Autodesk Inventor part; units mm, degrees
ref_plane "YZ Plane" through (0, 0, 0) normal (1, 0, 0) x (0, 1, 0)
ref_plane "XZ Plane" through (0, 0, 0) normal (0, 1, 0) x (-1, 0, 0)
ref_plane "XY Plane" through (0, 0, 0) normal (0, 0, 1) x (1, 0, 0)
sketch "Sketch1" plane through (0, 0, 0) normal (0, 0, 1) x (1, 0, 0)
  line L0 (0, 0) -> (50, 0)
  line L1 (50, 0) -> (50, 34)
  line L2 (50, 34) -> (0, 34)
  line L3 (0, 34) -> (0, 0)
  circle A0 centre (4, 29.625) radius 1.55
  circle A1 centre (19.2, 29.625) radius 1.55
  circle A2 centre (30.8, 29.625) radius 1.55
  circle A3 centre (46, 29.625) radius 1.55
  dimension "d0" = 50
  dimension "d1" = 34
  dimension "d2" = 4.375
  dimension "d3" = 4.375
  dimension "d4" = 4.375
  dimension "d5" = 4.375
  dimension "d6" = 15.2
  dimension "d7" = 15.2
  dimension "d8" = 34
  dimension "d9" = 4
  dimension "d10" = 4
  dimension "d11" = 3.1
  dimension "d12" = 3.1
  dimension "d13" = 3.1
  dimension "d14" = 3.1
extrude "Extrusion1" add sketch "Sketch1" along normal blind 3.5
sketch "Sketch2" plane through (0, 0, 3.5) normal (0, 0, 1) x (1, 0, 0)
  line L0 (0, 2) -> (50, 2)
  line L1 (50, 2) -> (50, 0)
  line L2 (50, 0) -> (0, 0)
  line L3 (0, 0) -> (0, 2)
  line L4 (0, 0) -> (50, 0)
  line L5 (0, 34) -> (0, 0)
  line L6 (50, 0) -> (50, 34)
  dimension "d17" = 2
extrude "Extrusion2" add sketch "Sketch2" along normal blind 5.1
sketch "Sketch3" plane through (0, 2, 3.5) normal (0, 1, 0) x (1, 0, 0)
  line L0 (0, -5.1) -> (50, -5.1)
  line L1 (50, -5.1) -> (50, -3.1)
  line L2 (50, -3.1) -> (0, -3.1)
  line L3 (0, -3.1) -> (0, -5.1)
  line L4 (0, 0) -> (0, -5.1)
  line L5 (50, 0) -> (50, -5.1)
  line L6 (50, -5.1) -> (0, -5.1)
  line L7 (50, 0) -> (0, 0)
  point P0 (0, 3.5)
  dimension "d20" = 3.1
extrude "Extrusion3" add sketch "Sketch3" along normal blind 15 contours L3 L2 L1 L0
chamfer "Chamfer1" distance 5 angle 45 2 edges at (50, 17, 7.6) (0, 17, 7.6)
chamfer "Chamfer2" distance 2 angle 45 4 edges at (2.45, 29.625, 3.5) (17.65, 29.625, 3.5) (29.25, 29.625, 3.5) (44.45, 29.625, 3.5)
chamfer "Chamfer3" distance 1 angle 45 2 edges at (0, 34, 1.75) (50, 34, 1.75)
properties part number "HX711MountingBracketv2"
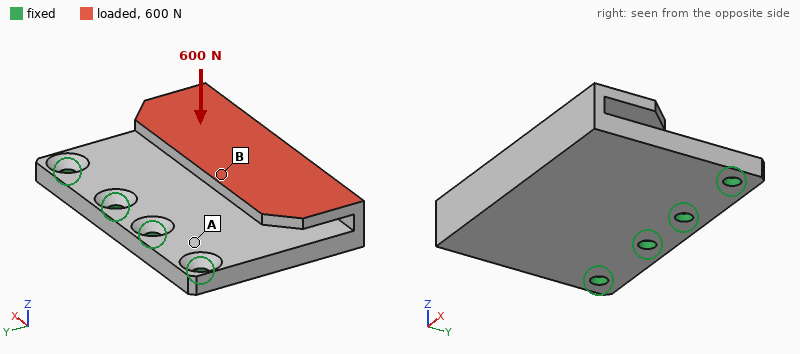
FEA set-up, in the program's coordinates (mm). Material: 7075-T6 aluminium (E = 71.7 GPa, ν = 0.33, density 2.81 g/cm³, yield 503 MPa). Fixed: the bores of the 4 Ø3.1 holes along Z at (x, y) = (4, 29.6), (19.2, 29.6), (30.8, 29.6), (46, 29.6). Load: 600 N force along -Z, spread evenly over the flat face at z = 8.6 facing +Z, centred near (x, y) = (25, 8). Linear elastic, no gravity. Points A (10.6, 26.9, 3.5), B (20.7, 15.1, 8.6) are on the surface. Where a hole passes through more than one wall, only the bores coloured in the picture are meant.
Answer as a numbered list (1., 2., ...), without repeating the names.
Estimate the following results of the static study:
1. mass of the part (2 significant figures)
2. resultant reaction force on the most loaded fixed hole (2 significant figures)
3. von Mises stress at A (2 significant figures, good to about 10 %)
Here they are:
1. 22 g
2. 200 N
3. 98 MPa
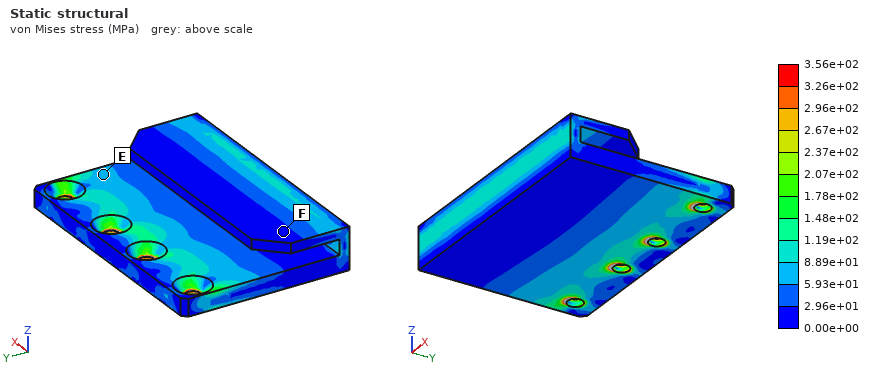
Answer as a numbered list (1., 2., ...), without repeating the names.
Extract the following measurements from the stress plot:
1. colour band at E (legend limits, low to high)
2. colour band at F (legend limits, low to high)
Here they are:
1. 5.93e+01 to 8.89e+01 MPa
2. 0.00e+00 to 2.96e+01 MPa
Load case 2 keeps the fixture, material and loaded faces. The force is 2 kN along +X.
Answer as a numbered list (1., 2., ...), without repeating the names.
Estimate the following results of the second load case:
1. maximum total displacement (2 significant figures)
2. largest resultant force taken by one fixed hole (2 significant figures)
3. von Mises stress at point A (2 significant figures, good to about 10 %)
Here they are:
1. 0.44 mm
2. 1.1 kN
3. 83 MPa
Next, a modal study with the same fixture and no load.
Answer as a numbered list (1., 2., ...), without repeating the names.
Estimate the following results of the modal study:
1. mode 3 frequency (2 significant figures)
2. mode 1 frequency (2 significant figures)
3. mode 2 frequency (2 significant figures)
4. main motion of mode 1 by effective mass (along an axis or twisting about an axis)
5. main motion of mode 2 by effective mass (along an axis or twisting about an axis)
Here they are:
1. 4500 Hz
2. 1800 Hz
3. 3400 Hz
4. along Z
5. twisting about Y
